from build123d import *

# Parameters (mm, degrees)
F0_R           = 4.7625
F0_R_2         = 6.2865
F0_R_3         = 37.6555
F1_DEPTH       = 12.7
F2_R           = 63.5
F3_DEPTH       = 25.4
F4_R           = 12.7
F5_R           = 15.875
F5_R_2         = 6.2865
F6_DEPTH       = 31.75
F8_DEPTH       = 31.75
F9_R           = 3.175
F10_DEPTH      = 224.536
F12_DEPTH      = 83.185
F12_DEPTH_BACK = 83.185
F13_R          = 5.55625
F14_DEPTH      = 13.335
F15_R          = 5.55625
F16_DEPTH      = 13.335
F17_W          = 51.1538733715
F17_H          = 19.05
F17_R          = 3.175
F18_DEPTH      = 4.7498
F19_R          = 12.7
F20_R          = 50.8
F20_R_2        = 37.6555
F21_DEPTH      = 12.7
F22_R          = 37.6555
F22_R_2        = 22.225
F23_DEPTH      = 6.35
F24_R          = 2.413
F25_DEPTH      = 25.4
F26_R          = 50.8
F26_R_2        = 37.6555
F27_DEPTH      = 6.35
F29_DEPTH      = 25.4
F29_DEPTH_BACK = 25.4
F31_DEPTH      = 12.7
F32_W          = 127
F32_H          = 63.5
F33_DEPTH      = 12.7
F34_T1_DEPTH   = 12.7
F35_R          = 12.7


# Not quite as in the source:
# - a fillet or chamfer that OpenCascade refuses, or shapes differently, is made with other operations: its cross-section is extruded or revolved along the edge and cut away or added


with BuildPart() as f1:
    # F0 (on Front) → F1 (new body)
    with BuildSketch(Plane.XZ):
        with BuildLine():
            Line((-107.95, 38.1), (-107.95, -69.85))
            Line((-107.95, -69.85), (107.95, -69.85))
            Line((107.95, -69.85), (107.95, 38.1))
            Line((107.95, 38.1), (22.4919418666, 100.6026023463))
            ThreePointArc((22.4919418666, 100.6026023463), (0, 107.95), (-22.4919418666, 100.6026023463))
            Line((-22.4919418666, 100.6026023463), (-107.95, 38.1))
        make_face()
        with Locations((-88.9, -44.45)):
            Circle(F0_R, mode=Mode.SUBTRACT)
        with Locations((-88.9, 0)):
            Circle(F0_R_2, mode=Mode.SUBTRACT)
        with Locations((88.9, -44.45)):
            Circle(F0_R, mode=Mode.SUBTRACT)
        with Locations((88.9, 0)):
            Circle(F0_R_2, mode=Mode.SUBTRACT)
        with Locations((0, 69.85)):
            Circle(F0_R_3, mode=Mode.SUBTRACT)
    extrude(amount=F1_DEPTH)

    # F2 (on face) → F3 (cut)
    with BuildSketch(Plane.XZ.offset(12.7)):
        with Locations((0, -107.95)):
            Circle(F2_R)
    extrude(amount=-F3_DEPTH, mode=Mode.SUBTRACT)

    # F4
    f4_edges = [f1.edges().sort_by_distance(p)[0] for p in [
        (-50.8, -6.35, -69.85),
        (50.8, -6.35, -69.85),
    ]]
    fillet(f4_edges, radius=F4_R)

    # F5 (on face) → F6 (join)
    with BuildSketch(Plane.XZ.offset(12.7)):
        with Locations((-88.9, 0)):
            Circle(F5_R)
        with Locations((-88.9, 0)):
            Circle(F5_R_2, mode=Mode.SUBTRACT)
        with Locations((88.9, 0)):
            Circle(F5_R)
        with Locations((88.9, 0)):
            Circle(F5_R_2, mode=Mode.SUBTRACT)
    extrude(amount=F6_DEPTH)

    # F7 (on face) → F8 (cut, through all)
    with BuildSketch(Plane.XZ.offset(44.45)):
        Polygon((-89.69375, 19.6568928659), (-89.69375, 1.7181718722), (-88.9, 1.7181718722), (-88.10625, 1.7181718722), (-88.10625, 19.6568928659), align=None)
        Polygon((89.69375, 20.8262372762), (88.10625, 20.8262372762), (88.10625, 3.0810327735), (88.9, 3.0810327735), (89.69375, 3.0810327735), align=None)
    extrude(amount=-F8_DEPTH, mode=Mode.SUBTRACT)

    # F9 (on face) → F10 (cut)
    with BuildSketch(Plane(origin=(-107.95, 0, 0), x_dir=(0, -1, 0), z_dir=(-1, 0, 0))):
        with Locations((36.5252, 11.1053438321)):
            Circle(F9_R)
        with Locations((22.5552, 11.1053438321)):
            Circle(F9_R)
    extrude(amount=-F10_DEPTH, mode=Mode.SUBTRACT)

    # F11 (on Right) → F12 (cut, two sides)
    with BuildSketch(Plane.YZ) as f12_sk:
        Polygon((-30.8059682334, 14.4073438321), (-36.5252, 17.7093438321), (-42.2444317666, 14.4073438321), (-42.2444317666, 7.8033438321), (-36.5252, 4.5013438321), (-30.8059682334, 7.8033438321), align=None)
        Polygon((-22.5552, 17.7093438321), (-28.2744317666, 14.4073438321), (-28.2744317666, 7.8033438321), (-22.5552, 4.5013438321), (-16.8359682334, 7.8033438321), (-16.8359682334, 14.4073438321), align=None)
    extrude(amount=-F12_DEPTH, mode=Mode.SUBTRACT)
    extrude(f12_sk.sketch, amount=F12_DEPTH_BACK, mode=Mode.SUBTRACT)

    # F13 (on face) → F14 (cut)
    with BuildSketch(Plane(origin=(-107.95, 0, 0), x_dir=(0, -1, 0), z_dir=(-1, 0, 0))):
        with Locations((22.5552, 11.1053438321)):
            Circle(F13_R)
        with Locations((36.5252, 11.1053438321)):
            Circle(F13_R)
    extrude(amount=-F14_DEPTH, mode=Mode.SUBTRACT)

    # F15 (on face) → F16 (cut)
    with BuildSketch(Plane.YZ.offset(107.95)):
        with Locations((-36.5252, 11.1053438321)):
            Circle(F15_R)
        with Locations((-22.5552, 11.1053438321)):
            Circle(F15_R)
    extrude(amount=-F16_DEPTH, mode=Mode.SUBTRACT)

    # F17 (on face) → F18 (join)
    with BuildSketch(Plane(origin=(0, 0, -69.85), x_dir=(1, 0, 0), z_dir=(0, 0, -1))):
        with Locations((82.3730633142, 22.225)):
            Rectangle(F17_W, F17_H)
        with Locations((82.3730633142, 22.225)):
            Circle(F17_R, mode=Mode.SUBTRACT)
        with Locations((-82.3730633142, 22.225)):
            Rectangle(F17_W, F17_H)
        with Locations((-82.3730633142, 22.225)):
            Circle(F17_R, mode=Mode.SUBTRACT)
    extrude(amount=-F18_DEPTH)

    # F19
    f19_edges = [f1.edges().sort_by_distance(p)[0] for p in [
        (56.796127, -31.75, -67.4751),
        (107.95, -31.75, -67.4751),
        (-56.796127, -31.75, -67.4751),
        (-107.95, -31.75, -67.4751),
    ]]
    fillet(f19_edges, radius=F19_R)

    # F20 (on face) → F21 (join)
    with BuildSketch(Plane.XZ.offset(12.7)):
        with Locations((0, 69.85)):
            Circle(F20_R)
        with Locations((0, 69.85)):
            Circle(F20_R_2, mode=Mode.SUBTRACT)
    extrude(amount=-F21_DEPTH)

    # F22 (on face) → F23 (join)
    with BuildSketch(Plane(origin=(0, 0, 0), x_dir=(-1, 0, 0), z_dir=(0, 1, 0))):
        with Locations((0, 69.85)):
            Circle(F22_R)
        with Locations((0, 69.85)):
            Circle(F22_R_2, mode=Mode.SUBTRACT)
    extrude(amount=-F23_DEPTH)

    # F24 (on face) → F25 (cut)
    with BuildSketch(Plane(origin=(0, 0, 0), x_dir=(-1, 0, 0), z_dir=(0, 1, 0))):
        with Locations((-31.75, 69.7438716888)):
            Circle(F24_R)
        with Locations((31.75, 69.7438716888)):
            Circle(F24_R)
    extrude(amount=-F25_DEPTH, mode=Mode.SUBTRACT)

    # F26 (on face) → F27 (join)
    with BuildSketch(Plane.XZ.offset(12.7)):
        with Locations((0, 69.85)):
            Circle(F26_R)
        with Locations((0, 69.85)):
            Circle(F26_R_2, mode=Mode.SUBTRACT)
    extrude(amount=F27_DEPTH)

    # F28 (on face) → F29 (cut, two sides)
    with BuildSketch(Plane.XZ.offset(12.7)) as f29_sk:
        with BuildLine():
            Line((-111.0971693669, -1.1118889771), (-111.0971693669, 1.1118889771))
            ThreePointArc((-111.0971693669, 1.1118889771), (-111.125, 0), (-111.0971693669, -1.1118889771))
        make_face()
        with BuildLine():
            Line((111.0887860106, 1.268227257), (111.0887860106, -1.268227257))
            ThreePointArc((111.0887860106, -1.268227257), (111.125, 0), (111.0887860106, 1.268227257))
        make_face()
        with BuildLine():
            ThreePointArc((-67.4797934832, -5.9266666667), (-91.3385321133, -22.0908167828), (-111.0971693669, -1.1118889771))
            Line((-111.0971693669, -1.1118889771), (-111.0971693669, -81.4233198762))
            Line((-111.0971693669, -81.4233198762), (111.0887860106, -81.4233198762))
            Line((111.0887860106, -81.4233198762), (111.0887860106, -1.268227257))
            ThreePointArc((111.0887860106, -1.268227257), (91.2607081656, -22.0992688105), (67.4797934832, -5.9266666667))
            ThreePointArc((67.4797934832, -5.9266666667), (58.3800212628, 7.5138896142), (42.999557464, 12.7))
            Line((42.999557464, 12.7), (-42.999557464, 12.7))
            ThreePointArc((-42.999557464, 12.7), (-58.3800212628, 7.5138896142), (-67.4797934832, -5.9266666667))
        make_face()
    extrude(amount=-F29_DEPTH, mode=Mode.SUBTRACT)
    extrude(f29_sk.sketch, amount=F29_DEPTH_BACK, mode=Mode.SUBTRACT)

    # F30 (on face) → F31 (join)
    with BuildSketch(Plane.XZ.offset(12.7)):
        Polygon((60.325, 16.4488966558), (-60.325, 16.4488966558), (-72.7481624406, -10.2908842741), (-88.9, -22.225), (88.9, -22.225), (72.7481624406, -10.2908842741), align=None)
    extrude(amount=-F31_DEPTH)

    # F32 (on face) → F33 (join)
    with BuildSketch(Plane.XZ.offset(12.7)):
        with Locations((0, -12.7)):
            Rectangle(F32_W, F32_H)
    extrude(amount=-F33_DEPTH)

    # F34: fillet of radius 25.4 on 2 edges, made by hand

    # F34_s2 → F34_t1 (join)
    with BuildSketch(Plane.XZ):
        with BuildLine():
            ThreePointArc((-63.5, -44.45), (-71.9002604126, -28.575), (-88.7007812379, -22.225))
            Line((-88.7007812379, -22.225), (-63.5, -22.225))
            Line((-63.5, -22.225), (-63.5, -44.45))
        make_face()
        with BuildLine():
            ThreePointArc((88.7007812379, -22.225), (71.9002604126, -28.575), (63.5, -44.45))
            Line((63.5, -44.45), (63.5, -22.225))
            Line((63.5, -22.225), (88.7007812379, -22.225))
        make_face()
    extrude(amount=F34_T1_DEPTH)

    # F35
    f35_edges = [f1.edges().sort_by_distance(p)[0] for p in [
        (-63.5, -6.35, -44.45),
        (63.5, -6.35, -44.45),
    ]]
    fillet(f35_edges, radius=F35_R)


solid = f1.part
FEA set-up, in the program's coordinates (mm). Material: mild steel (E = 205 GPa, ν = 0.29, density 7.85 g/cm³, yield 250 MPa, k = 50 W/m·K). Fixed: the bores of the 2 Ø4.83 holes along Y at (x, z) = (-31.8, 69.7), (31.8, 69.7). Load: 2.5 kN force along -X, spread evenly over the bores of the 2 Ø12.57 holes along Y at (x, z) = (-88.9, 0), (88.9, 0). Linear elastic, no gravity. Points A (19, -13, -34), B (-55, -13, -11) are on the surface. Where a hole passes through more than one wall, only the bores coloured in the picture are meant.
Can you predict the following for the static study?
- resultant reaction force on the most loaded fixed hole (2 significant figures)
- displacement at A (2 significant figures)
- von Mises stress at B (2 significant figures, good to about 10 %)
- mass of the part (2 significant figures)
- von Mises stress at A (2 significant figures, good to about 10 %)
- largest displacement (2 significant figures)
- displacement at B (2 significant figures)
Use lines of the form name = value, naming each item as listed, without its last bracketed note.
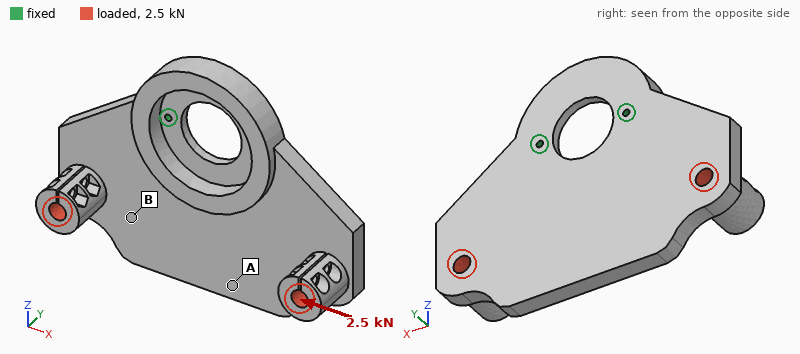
resultant reaction force on the most loaded fixed hole = 3.0 kN
displacement at A = 15 µm
von Mises stress at B = 8.7 MPa
mass of the part = 2.7 kg
von Mises stress at A = 4.2 MPa
largest displacement = 53 µm
displacement at B = 21 µm
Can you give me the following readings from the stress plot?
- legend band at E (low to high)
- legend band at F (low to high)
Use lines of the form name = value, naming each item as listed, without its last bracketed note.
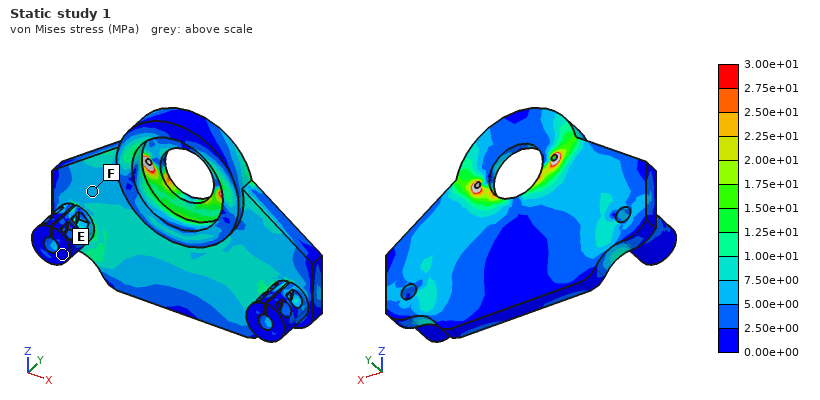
legend band at E = 0.00e+00 to 2.50e+00 MPa
legend band at F = 5.00e+00 to 7.50e+00 MPa
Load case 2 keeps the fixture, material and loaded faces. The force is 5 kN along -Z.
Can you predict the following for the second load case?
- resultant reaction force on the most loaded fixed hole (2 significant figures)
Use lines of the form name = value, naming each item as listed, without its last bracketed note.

resultant reaction force on the most loaded fixed hole = 2.6 kN
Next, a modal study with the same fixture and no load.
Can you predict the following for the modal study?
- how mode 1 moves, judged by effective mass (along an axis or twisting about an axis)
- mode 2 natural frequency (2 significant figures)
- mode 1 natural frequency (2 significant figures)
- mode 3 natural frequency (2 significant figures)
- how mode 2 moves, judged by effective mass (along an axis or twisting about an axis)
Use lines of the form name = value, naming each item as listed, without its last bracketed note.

how mode 1 moves, judged by effective mass = along Y
mode 2 natural frequency = 670 Hz
mode 1 natural frequency = 320 Hz
mode 3 natural frequency = 1400 Hz
how mode 2 moves, judged by effective mass = twisting about Z
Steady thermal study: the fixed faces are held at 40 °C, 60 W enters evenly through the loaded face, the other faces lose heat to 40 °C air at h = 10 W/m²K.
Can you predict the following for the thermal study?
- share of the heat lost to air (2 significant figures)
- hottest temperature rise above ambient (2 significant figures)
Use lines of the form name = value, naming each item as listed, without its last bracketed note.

share of the heat lost to air = 44 %
hottest temperature rise above ambient = 71 K
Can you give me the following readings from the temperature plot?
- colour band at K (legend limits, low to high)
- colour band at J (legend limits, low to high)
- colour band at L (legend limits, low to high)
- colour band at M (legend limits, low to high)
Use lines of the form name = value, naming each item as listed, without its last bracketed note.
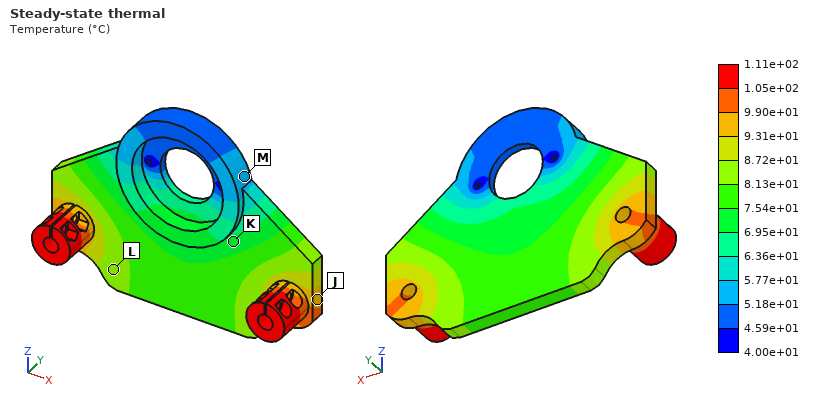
colour band at K = 6.95e+01 to 7.54e+01 °C
colour band at J = 9.31e+01 to 9.90e+01 °C
colour band at L = 8.13e+01 to 8.72e+01 °C
colour band at M = 5.18e+01 to 5.77e+01 °C
